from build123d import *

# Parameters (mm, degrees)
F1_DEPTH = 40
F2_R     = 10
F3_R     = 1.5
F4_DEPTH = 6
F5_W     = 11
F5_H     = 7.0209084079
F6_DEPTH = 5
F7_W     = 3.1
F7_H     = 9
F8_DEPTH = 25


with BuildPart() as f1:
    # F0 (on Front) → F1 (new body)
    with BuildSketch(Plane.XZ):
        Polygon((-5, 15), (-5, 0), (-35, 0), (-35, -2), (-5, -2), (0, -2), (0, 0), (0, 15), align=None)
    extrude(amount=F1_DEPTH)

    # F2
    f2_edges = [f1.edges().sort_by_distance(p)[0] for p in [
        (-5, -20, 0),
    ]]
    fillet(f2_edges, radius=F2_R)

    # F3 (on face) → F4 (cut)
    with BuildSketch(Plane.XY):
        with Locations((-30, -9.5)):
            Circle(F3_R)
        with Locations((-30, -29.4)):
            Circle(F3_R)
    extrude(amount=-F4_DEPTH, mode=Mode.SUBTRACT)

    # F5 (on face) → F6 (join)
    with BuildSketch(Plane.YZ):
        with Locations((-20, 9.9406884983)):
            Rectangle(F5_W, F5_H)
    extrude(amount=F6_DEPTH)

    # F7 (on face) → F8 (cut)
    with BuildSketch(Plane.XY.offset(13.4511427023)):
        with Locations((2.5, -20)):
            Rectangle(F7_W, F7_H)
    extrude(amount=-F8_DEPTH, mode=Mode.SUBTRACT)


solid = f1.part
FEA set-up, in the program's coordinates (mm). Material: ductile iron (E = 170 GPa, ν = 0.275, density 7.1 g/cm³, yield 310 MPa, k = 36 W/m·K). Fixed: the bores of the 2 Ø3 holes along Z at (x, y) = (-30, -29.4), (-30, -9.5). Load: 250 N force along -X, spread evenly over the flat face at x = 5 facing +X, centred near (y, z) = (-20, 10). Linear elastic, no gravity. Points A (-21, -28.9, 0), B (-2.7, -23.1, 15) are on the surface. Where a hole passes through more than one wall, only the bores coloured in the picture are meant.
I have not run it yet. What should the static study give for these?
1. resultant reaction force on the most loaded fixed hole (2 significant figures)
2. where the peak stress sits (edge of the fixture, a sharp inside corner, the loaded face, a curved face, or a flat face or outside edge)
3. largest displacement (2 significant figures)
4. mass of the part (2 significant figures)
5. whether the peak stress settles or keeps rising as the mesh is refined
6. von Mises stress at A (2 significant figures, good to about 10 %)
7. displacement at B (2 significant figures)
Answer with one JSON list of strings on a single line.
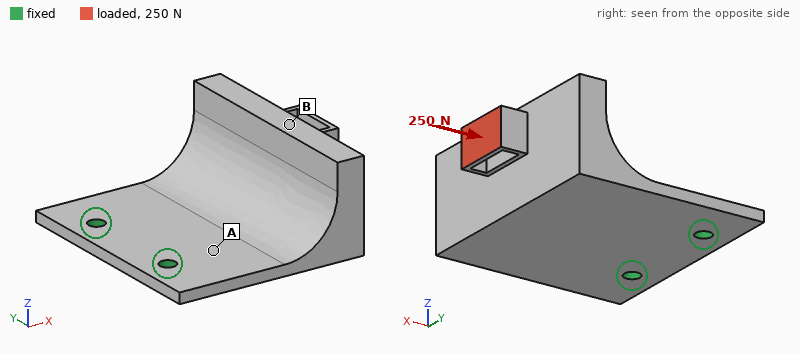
["130 N", "edge of the fixture", "0.34 mm", "48 g", "keeps rising", "96 MPa", "0.27 mm"]
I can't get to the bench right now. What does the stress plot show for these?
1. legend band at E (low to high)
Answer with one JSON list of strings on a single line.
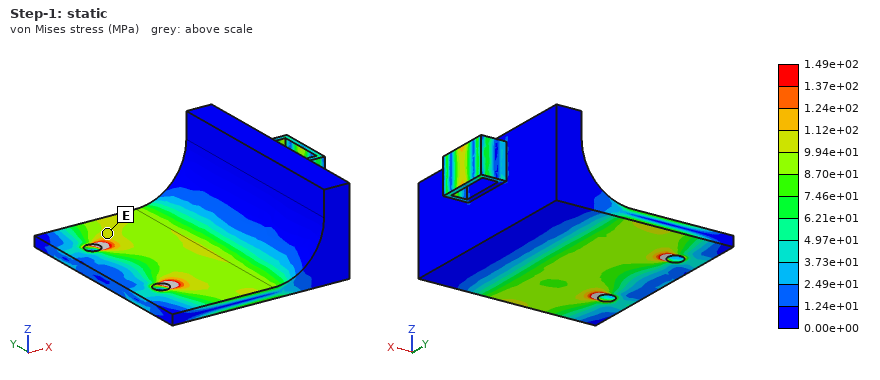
["9.94e+01 to 1.12e+02 MPa"]
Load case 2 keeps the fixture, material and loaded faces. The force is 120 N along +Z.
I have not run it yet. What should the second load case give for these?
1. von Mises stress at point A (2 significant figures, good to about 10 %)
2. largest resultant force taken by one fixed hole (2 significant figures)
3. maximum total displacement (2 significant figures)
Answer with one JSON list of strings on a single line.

["100 MPa", "63 N", "0.39 mm"]
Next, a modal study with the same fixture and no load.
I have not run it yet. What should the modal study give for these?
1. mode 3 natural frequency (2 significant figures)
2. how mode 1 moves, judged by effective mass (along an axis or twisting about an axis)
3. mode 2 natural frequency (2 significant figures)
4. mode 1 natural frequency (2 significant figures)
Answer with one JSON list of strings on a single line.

["4700 Hz", "along Z", "1900 Hz", "660 Hz"]
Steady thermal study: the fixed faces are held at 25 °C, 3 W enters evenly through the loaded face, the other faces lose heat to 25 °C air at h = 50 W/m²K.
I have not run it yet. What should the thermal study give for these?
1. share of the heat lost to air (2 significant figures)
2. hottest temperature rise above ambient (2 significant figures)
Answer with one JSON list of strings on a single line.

["65 %", "49 K"]
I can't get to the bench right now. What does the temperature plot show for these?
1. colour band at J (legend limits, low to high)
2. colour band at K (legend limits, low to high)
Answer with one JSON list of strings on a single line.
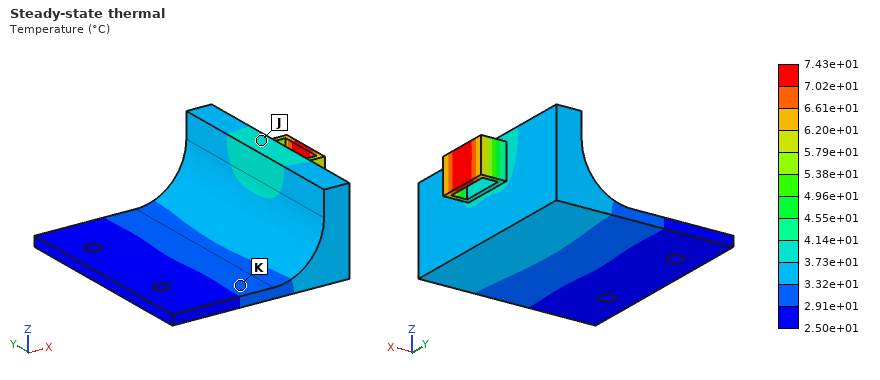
["3.73e+01 to 4.14e+01 °C", "2.91e+01 to 3.32e+01 °C"]
